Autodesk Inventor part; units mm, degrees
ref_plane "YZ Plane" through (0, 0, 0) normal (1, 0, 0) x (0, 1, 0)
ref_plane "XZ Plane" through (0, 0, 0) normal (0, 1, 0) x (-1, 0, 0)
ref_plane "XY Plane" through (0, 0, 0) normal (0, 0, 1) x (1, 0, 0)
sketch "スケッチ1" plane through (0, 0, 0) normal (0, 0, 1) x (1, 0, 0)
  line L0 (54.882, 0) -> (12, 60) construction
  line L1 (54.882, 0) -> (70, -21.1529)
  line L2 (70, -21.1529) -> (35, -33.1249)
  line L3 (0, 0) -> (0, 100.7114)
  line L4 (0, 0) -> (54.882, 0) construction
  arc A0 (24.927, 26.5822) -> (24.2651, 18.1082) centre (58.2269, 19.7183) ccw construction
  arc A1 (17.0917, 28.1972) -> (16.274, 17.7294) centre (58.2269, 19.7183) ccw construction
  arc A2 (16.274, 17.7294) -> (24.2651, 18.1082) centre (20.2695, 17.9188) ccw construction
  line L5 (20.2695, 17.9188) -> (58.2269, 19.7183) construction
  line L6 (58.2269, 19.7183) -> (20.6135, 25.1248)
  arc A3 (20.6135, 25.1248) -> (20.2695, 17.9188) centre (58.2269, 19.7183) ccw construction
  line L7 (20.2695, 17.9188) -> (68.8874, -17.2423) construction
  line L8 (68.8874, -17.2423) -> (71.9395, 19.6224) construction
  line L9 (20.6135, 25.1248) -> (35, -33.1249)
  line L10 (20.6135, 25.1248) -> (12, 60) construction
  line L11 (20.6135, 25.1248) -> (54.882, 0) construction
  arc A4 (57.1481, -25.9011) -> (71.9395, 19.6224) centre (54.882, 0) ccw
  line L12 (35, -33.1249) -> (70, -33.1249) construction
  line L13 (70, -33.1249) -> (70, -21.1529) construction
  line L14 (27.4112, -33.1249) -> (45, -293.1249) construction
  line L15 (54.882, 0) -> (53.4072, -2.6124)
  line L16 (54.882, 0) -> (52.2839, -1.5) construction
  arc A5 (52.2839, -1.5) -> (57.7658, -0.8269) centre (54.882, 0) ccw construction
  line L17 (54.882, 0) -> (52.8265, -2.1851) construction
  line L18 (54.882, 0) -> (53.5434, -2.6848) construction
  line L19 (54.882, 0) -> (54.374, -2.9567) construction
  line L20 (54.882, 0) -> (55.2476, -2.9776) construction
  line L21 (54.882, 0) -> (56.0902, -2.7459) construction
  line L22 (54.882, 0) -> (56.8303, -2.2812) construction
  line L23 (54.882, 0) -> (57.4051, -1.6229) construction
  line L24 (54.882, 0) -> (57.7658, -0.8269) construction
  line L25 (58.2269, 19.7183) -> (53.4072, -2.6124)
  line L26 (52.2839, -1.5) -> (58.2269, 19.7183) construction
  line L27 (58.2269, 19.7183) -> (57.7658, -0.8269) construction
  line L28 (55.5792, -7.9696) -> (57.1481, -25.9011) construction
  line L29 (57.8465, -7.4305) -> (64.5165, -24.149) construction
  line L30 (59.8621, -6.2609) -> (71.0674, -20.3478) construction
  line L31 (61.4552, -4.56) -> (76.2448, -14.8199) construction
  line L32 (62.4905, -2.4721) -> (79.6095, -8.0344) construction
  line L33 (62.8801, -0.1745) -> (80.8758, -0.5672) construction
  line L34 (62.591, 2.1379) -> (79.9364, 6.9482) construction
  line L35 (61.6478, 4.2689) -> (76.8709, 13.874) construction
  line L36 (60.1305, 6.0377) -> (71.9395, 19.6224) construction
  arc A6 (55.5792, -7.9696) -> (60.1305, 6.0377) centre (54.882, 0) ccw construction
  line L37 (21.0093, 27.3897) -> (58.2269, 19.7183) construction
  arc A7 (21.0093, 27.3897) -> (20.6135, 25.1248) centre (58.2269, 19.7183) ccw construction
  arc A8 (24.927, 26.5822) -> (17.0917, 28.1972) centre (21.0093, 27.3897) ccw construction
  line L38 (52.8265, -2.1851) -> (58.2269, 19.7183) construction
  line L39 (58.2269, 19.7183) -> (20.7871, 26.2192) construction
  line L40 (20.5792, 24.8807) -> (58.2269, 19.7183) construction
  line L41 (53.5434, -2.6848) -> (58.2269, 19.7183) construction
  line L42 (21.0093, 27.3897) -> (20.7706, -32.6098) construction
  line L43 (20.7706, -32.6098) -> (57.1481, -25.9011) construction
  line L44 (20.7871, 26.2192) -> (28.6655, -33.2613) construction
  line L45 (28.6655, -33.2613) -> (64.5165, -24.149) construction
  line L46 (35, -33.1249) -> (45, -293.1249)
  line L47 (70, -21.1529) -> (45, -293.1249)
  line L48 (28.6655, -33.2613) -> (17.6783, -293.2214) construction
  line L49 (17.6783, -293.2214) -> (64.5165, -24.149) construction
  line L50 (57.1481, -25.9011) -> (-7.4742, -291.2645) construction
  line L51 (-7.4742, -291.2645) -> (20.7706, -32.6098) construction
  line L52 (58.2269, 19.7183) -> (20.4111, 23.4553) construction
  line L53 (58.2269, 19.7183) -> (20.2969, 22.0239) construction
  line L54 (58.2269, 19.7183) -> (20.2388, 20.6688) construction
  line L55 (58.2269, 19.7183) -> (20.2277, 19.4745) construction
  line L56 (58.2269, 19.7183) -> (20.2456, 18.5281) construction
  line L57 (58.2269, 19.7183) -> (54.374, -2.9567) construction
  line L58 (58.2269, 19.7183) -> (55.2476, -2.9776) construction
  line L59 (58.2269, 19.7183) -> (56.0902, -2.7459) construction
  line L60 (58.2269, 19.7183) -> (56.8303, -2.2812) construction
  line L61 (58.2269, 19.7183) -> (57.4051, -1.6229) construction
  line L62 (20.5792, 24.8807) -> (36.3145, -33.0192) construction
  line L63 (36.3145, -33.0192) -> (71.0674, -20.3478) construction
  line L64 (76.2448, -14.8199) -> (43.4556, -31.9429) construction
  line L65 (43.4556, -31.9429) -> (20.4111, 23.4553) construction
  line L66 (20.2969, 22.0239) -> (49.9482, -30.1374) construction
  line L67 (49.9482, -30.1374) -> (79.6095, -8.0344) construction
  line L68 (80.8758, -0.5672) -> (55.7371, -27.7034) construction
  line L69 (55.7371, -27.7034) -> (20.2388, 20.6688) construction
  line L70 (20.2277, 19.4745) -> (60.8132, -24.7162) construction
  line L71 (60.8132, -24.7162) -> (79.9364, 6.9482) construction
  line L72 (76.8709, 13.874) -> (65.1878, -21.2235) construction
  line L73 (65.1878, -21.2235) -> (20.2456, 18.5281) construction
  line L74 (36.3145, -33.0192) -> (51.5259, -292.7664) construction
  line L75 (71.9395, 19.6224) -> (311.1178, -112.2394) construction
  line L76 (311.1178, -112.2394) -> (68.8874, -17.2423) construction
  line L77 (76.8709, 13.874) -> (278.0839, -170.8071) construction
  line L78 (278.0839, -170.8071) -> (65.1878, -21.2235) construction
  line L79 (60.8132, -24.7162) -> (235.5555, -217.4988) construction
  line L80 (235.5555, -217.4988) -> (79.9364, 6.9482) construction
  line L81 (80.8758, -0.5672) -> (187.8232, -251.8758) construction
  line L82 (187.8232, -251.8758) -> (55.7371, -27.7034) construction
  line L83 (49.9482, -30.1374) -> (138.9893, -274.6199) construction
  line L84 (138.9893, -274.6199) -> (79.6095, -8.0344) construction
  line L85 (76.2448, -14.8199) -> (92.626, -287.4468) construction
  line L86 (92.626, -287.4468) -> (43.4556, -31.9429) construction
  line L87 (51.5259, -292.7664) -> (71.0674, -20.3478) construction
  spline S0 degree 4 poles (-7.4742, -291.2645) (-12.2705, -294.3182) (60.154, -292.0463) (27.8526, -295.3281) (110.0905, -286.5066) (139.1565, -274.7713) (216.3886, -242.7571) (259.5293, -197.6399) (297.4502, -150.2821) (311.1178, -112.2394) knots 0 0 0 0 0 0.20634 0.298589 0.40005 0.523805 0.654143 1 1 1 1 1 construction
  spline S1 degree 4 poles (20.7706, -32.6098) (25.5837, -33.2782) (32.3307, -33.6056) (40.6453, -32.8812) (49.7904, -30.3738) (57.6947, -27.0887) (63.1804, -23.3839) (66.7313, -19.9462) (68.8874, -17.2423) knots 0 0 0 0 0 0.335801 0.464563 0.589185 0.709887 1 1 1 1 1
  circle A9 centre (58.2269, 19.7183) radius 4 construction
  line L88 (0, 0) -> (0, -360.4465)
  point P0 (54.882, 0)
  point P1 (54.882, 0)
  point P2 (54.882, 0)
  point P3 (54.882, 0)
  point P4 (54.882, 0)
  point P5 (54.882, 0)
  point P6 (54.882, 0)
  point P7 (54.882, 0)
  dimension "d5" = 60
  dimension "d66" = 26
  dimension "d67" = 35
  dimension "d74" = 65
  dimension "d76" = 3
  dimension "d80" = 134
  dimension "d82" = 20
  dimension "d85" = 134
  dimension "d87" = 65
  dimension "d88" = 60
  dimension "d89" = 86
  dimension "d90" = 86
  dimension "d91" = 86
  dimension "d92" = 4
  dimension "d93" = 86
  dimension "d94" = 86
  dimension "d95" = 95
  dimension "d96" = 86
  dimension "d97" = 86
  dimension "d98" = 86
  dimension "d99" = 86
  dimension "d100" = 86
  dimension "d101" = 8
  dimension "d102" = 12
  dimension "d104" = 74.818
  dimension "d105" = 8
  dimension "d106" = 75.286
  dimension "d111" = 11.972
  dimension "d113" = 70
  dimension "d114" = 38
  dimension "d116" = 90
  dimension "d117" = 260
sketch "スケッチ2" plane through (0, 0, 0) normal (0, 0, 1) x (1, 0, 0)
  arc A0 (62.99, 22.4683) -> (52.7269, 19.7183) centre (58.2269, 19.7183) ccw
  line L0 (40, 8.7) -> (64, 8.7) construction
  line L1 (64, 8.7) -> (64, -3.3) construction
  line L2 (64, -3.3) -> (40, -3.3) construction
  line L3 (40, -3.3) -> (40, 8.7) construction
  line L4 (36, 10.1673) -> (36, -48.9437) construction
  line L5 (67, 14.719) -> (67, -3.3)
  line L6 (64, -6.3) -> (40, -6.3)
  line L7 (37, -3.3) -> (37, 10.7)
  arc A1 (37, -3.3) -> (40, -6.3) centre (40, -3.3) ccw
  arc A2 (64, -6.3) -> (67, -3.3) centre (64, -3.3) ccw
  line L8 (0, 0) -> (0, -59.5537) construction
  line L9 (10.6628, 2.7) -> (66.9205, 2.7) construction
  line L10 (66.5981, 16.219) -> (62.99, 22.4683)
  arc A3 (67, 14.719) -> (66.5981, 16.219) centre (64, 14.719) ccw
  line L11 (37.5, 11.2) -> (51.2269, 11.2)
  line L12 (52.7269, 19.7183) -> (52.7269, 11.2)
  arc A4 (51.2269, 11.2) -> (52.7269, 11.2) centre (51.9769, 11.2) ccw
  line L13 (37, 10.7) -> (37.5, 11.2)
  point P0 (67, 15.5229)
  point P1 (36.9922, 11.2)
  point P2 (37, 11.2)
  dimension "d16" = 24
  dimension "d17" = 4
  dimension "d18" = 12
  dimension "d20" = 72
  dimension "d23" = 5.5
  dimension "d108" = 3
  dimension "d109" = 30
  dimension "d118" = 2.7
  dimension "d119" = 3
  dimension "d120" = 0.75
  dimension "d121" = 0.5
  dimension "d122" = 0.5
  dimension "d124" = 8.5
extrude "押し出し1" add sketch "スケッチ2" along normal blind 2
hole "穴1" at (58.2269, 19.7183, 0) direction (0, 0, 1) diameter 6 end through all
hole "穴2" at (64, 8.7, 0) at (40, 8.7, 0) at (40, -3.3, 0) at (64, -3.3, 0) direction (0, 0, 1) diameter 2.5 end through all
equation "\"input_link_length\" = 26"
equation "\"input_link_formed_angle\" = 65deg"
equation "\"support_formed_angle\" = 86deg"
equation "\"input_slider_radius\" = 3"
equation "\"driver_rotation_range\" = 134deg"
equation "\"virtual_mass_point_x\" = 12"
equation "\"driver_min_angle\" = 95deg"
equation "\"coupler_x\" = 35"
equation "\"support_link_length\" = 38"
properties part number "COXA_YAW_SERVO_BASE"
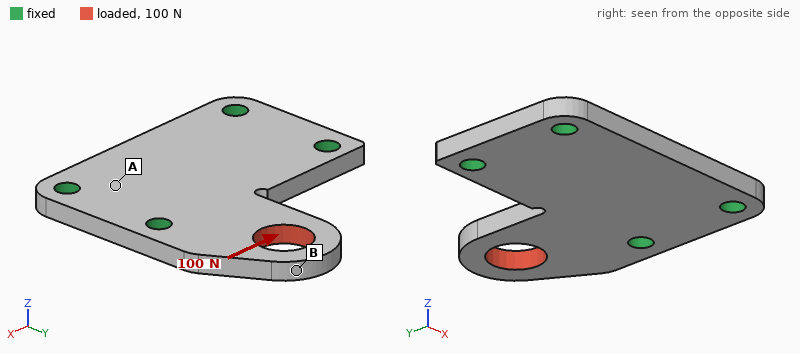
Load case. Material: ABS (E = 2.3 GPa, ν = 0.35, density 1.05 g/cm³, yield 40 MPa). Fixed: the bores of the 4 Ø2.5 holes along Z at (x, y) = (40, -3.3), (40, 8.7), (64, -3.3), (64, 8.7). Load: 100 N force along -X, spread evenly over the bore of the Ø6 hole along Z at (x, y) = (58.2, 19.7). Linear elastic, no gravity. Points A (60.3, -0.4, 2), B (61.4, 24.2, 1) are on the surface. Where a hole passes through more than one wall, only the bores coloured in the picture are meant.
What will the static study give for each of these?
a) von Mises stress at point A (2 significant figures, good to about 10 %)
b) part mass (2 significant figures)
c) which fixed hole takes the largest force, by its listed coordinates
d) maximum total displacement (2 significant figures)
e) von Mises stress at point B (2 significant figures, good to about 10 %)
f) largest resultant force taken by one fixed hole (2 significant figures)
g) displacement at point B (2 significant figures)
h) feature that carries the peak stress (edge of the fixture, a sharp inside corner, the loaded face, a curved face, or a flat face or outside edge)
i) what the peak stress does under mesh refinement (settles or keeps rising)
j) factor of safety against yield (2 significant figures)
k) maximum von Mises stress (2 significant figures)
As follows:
3.3 MPa
1.3 g
(64, 8.7)
0.23 mm
8.5 MPa
110 N
0.22 mm
a curved face
settles
0.96
42 MPa
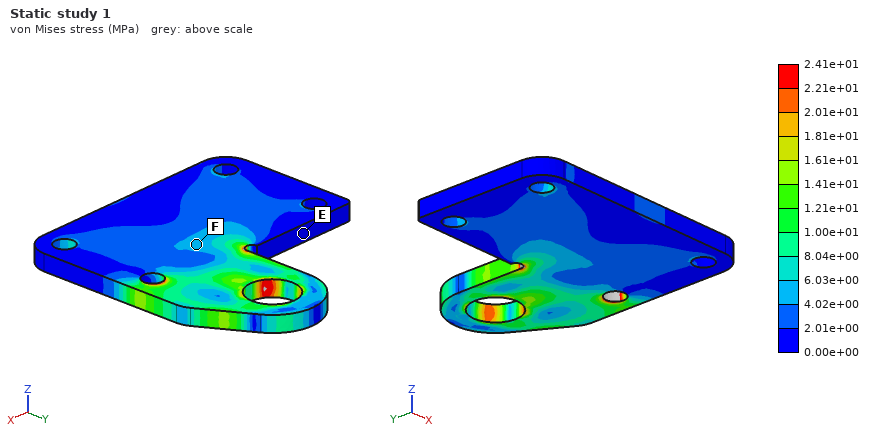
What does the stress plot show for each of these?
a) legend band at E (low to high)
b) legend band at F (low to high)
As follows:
0.00e+00 to 2.01e+00 MPa
4.02e+00 to 6.03e+00 MPa
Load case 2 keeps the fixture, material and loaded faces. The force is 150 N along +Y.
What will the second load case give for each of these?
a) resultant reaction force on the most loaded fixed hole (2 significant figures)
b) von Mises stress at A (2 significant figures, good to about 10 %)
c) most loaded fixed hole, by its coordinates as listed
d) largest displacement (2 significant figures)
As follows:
83 N
3.6 MPa
(64, 8.7)
0.11 mm
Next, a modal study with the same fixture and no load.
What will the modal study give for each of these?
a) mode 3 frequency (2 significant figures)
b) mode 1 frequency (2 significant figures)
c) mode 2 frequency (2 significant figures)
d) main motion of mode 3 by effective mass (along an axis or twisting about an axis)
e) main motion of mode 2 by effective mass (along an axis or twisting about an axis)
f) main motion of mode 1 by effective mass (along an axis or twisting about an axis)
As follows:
6100 Hz
2200 Hz
4900 Hz
along Z
along Z
along Z
